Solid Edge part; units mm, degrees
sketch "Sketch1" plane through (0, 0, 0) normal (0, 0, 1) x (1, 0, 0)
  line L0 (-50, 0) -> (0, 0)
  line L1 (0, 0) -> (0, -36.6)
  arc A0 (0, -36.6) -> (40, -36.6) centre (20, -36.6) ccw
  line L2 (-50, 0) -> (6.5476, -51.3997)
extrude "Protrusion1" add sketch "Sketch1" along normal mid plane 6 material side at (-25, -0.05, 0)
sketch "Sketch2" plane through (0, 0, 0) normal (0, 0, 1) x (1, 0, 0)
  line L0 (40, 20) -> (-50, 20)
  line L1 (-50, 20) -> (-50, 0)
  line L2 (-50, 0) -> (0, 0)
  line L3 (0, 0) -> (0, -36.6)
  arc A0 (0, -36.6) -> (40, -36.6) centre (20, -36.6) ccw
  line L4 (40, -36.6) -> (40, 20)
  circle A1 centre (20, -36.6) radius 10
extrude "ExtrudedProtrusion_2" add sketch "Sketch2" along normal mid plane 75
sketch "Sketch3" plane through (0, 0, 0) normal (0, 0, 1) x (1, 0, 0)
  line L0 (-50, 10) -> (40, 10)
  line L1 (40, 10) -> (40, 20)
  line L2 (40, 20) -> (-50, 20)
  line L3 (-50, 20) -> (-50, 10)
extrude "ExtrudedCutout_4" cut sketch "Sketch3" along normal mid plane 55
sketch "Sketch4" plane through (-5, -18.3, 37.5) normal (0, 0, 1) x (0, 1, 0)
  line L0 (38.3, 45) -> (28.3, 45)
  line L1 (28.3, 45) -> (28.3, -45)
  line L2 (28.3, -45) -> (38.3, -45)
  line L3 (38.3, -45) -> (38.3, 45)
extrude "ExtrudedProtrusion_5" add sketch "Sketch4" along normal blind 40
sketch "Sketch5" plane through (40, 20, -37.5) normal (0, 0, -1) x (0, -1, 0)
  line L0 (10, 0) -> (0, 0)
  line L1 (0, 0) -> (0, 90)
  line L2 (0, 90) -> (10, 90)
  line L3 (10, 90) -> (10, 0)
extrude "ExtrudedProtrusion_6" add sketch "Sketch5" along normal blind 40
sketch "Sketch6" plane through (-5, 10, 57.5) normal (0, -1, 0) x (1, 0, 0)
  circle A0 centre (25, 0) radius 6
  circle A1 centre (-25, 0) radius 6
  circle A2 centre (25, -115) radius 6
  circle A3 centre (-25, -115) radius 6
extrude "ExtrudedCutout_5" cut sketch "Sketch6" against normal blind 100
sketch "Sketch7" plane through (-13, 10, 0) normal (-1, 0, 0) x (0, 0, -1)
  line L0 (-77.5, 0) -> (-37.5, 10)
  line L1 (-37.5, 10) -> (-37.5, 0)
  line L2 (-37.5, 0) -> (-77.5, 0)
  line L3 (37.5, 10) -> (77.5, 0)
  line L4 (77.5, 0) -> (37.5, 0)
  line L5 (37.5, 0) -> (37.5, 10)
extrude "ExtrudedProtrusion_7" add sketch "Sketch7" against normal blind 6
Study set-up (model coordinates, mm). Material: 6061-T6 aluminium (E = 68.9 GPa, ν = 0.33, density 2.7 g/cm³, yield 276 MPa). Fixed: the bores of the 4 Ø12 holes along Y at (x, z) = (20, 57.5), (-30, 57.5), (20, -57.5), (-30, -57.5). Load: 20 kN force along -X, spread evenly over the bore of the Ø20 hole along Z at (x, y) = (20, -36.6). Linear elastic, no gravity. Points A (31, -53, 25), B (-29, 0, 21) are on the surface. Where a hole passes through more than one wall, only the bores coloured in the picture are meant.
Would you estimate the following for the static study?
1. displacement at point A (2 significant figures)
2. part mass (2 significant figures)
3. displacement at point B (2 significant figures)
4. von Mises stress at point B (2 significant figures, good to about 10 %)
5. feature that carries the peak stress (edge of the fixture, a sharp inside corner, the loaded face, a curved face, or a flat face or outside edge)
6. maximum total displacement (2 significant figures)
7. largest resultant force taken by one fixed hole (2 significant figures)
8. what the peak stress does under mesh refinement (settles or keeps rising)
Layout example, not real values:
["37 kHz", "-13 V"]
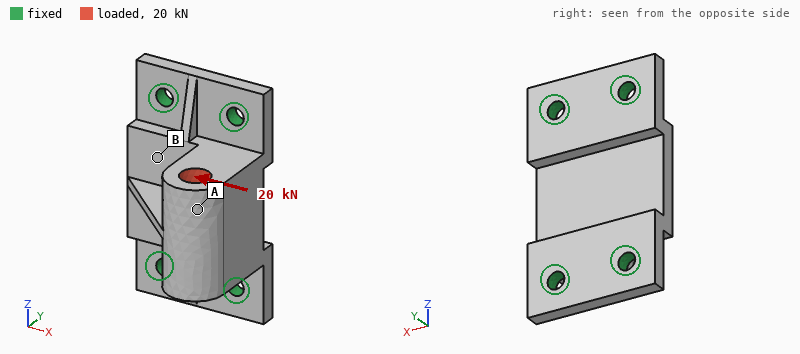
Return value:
["0.36 mm", "800 g", "0.11 mm", "49 MPa", "edge of the fixture", "0.37 mm", "18 kN", "keeps rising"]
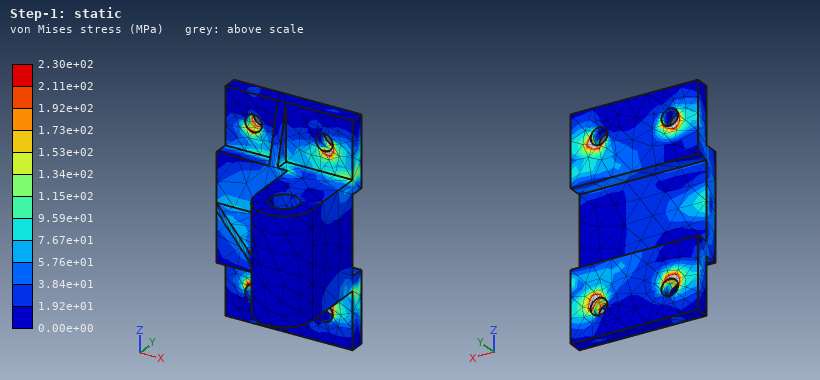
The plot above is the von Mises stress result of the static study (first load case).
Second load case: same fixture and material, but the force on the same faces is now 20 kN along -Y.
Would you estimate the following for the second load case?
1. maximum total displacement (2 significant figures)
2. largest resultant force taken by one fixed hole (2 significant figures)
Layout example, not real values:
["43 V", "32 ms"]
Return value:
["0.13 mm", "12 kN"]
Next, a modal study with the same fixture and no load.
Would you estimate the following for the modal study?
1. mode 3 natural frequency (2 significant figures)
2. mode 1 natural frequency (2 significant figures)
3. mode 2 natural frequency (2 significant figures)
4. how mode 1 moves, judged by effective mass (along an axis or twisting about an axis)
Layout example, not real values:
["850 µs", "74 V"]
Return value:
["4200 Hz", "2400 Hz", "4200 Hz", "along X"]
